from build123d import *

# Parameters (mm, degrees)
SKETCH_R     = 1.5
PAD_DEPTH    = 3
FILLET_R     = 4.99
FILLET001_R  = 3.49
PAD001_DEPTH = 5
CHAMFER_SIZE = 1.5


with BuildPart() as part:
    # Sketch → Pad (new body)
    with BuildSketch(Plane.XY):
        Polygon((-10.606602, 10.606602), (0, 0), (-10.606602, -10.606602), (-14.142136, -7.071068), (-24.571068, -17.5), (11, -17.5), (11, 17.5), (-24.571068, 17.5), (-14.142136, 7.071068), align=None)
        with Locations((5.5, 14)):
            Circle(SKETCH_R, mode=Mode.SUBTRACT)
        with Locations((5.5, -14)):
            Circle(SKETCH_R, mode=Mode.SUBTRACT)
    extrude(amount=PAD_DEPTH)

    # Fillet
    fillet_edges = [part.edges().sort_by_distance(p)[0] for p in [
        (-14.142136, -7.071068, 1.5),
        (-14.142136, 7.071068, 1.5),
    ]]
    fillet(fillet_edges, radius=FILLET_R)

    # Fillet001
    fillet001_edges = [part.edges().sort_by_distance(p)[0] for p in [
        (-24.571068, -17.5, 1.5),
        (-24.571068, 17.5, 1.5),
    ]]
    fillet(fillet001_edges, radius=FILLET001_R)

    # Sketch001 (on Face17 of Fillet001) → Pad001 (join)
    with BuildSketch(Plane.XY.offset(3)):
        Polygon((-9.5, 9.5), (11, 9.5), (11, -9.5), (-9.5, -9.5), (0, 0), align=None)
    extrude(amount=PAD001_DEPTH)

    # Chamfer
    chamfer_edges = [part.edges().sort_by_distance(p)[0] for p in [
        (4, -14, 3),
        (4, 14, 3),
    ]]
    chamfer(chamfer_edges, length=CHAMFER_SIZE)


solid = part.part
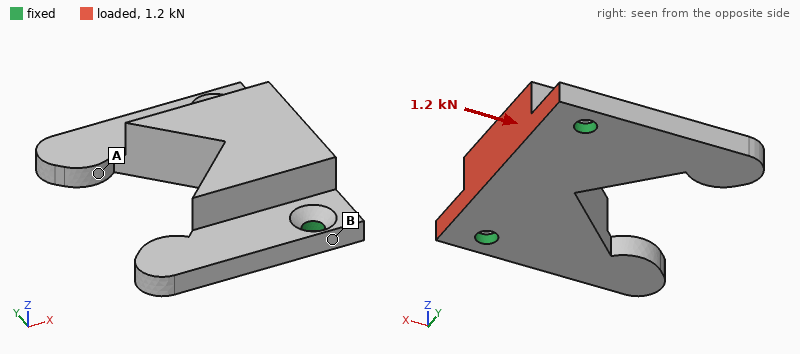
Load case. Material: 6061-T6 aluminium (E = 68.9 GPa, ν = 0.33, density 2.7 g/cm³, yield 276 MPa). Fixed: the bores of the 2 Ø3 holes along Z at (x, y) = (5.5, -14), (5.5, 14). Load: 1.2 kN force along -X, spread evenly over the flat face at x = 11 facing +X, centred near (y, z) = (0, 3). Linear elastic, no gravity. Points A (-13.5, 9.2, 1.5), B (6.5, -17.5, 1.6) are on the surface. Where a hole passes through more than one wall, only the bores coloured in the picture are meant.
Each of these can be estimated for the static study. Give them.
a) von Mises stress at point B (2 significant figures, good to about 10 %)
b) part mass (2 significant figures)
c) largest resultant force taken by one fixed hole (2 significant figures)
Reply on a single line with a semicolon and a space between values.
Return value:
45 MPa; 10 g; 600 N
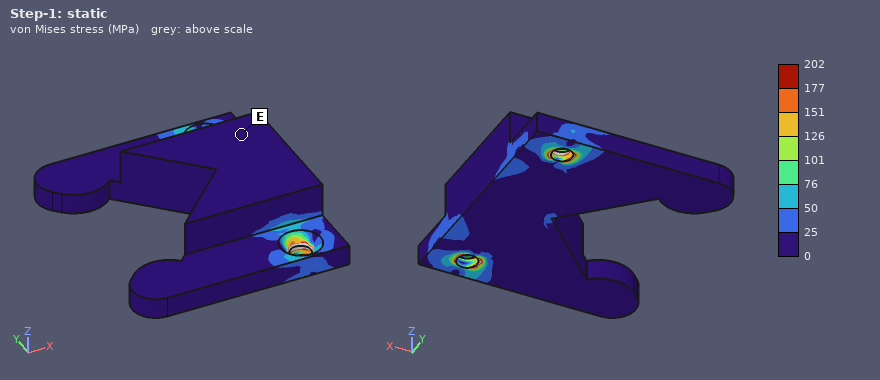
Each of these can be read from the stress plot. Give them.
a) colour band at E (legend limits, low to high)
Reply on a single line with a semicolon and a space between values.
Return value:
0 to 25 MPa
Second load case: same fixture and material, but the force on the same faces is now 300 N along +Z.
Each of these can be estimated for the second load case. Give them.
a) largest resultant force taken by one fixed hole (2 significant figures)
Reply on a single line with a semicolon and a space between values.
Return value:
200 N
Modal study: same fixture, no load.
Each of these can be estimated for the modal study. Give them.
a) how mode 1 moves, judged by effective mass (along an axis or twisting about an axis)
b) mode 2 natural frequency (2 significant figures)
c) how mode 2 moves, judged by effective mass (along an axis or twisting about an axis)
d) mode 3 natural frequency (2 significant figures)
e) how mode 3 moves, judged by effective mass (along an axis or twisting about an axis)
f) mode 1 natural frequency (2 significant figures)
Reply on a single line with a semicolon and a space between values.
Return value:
along Z; 8500 Hz; twisting about X; 14 kHz; along X; 4300 Hz
